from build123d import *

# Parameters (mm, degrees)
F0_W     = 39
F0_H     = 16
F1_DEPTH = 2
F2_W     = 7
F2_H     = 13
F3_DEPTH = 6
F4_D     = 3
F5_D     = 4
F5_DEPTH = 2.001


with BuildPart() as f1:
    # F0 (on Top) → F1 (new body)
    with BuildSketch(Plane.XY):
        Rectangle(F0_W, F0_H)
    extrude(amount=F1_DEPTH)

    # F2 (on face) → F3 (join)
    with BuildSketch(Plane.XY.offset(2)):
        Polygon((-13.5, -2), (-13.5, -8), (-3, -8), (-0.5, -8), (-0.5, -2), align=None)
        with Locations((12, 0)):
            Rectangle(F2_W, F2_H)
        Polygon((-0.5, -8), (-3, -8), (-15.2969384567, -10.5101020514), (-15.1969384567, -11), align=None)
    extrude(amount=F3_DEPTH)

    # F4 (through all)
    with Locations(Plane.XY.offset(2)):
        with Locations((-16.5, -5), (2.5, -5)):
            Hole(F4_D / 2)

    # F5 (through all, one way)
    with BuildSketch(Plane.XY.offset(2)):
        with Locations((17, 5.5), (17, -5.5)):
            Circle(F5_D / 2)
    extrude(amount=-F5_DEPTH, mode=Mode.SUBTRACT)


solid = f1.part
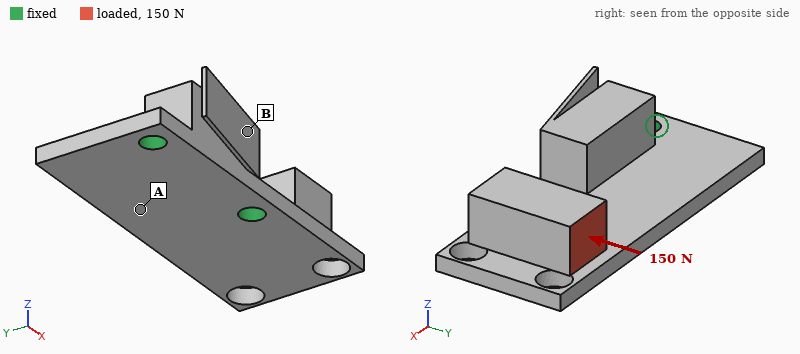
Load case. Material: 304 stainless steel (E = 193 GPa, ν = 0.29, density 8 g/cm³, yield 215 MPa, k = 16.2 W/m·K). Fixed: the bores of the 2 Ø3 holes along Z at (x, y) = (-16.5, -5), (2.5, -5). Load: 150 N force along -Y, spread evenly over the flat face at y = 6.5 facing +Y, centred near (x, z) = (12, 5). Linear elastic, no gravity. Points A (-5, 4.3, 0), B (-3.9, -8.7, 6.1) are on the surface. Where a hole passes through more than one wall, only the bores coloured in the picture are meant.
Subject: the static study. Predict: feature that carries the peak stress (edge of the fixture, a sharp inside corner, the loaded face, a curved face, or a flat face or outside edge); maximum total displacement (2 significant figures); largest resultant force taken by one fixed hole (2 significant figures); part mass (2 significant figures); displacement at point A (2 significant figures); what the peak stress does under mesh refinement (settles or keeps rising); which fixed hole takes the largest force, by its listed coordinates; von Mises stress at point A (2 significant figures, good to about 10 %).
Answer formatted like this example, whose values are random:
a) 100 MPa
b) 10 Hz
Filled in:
a) edge of the fixture
b) 18 µm
c) 210 N
d) 18 g
e) 2.9 µm
f) keeps rising
g) (2.5, -5)
h) 20 MPa
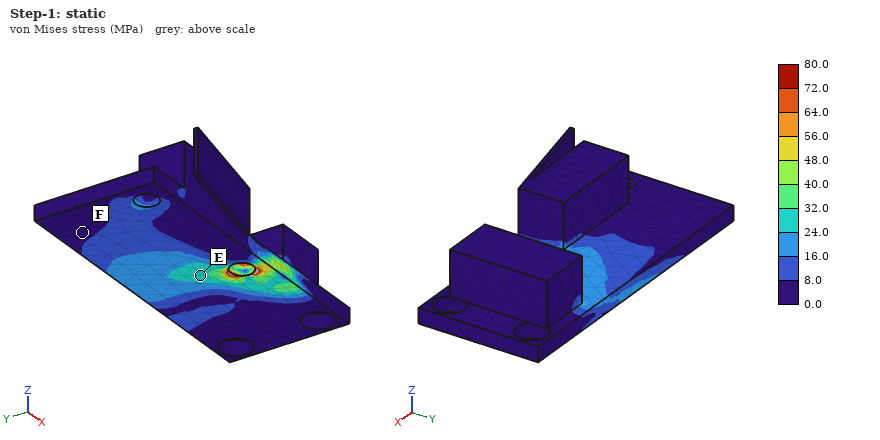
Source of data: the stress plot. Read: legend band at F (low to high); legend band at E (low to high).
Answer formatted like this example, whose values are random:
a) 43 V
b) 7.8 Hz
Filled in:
a) 0.0 to 8.0 MPa
b) 24.0 to 32.0 MPa
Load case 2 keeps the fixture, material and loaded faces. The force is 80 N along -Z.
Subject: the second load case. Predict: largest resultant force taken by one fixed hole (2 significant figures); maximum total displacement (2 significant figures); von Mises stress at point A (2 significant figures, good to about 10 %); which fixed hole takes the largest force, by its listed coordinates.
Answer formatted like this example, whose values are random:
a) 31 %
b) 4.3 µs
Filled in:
a) 97 N
b) 51 µm
c) 26 MPa
d) (2.5, -5)
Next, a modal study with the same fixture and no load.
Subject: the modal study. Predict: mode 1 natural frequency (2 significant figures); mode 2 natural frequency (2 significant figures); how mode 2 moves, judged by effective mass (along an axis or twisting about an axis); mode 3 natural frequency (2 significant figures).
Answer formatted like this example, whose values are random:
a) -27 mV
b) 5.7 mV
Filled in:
a) 2500 Hz
b) 3600 Hz
c) along Z
d) 7400 Hz
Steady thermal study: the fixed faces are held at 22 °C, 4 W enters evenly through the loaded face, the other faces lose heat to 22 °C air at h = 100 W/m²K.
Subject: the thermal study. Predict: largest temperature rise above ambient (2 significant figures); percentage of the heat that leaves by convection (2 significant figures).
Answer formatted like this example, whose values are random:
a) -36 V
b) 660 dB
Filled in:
a) 60 K
b) 67 %
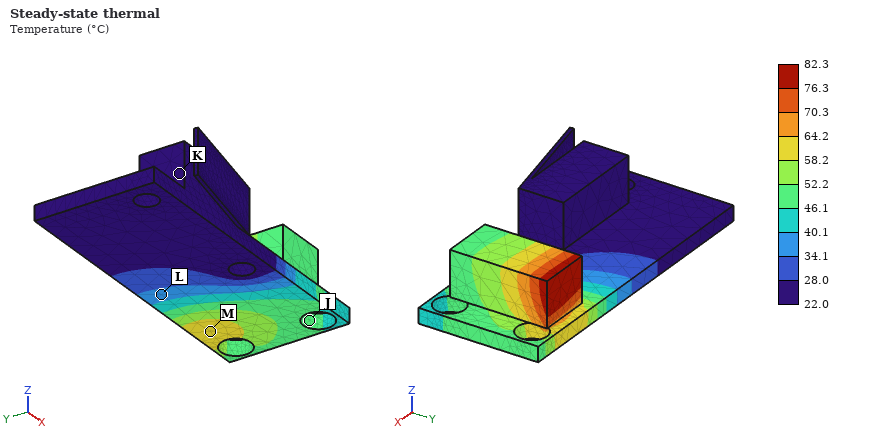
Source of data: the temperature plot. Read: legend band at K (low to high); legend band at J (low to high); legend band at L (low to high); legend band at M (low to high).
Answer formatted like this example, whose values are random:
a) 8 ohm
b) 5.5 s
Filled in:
a) 22.0 to 28.0 °C
b) 46.1 to 52.2 °C
c) 34.1 to 40.1 °C
d) 58.2 to 64.2 °C
